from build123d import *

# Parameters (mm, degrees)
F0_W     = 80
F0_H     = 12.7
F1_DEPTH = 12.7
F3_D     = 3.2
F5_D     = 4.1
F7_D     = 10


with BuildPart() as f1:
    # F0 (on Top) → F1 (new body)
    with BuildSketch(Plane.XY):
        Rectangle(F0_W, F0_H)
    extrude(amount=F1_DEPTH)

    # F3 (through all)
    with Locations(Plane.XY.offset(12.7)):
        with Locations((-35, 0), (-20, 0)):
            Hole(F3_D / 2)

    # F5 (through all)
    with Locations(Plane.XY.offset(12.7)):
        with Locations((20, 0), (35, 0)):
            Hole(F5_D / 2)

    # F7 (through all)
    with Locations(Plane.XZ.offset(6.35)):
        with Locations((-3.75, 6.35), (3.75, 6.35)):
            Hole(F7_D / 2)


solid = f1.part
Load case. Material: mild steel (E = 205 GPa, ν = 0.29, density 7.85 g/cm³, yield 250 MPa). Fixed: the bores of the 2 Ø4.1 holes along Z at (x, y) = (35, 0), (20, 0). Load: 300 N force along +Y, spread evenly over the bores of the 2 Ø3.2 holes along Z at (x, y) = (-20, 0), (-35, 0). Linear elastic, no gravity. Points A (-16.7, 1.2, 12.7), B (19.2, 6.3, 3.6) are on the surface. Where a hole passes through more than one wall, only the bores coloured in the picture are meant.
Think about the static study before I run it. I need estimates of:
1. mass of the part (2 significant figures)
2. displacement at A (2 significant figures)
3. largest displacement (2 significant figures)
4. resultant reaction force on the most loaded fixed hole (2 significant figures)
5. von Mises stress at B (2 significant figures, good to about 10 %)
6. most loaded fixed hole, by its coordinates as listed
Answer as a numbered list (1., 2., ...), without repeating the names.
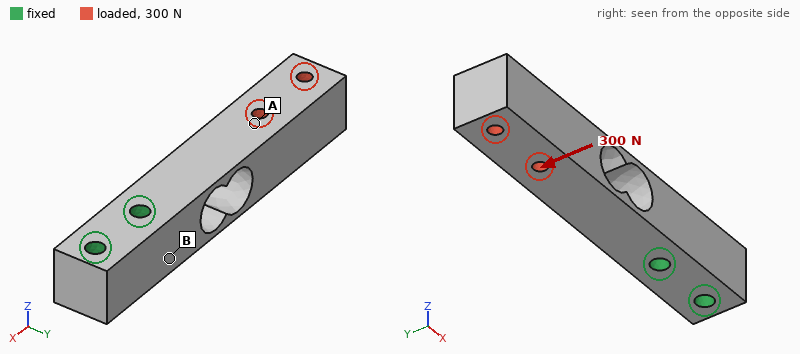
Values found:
1. 83 g
2. 42 µm
3. 90 µm
4. 750 N
5. 31 MPa
6. (20, 0)
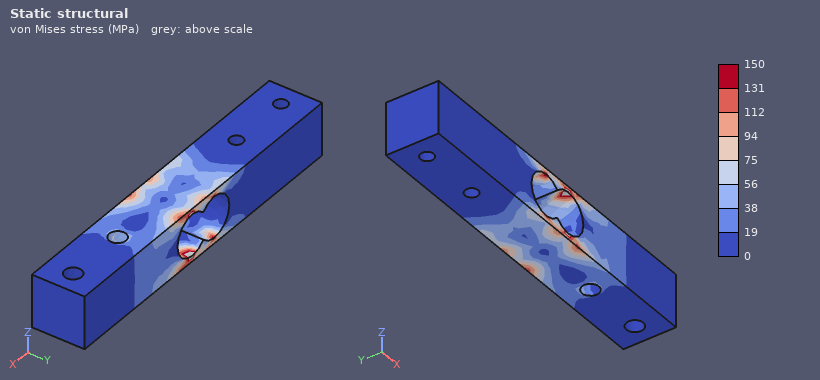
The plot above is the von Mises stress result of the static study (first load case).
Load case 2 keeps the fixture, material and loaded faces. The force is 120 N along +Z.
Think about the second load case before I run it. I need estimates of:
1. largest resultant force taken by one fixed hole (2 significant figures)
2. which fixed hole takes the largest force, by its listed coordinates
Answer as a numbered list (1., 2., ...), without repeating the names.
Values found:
1. 170 N
2. (20, 0)
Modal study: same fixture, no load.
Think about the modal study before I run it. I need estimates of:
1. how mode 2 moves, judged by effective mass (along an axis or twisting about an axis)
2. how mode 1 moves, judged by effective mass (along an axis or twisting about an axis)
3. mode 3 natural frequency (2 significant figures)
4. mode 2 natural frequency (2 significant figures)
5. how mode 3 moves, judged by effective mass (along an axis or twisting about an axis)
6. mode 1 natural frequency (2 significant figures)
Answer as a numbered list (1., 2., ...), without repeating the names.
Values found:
1. along Y
2. along Z
3. 7000 Hz
4. 1800 Hz
5. twisting about X
6. 1600 Hz
